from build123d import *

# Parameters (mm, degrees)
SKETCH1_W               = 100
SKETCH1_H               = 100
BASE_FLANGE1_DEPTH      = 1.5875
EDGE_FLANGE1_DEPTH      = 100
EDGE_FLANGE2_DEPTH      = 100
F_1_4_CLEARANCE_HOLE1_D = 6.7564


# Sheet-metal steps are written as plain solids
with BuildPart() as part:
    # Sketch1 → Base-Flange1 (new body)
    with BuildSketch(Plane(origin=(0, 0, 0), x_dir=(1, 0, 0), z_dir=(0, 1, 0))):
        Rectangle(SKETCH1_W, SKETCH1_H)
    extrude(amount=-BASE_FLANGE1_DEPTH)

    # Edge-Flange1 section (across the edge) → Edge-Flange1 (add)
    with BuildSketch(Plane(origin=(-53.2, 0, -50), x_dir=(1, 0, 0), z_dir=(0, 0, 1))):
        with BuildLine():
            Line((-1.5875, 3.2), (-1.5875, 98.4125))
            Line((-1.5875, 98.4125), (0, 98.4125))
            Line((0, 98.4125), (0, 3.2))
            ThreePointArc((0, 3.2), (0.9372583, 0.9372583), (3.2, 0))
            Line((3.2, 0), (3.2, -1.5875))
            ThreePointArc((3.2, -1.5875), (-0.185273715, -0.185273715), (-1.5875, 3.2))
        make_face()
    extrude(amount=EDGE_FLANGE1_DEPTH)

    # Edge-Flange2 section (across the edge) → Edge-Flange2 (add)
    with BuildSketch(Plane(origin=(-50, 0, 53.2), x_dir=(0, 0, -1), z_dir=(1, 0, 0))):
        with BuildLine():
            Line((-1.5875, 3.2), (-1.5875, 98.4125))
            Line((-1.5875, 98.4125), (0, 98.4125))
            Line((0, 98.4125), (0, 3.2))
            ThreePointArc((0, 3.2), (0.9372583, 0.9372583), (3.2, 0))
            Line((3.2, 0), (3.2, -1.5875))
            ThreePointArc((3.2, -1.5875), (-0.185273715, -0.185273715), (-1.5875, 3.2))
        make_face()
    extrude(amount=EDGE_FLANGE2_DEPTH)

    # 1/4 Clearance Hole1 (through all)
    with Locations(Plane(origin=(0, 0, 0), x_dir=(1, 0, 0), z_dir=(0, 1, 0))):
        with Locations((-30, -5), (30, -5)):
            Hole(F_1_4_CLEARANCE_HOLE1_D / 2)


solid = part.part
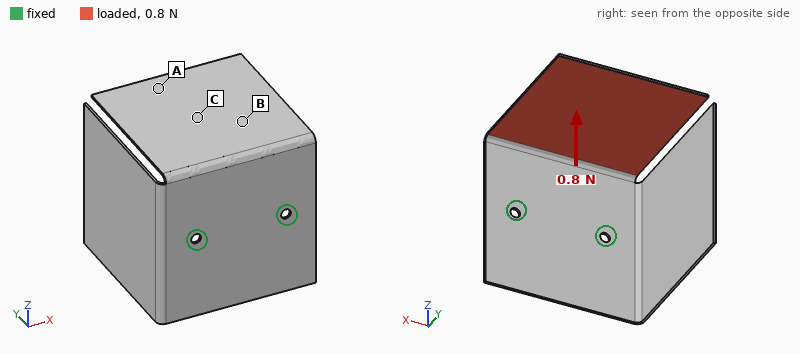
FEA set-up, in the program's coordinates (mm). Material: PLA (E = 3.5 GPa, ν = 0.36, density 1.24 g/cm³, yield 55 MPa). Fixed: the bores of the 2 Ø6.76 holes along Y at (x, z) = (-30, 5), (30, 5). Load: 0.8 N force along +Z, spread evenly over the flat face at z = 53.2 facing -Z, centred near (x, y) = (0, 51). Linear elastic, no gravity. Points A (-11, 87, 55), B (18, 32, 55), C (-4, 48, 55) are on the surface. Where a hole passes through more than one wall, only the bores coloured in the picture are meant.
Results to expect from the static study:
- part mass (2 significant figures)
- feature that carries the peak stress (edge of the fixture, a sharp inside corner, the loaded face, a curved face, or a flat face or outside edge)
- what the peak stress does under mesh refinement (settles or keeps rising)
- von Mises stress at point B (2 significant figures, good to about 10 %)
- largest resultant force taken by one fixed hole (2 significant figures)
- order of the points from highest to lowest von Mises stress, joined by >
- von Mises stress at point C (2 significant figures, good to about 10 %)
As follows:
59 g
a sharp inside corner
keeps rising
0.36 MPa
0.47 N
B > C > A
0.23 MPa
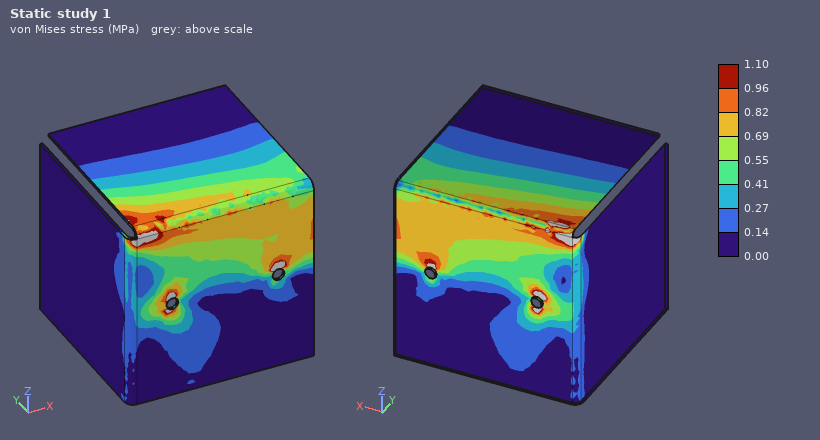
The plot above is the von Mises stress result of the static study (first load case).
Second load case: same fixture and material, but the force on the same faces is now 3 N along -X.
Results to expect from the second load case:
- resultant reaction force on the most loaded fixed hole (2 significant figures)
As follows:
3.5 N
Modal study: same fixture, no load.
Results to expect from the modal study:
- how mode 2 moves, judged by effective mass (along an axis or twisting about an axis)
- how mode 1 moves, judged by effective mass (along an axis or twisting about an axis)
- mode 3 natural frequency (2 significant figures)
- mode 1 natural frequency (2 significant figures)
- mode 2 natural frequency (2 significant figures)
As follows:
along X
along Z
45 Hz
28 Hz
33 Hz
